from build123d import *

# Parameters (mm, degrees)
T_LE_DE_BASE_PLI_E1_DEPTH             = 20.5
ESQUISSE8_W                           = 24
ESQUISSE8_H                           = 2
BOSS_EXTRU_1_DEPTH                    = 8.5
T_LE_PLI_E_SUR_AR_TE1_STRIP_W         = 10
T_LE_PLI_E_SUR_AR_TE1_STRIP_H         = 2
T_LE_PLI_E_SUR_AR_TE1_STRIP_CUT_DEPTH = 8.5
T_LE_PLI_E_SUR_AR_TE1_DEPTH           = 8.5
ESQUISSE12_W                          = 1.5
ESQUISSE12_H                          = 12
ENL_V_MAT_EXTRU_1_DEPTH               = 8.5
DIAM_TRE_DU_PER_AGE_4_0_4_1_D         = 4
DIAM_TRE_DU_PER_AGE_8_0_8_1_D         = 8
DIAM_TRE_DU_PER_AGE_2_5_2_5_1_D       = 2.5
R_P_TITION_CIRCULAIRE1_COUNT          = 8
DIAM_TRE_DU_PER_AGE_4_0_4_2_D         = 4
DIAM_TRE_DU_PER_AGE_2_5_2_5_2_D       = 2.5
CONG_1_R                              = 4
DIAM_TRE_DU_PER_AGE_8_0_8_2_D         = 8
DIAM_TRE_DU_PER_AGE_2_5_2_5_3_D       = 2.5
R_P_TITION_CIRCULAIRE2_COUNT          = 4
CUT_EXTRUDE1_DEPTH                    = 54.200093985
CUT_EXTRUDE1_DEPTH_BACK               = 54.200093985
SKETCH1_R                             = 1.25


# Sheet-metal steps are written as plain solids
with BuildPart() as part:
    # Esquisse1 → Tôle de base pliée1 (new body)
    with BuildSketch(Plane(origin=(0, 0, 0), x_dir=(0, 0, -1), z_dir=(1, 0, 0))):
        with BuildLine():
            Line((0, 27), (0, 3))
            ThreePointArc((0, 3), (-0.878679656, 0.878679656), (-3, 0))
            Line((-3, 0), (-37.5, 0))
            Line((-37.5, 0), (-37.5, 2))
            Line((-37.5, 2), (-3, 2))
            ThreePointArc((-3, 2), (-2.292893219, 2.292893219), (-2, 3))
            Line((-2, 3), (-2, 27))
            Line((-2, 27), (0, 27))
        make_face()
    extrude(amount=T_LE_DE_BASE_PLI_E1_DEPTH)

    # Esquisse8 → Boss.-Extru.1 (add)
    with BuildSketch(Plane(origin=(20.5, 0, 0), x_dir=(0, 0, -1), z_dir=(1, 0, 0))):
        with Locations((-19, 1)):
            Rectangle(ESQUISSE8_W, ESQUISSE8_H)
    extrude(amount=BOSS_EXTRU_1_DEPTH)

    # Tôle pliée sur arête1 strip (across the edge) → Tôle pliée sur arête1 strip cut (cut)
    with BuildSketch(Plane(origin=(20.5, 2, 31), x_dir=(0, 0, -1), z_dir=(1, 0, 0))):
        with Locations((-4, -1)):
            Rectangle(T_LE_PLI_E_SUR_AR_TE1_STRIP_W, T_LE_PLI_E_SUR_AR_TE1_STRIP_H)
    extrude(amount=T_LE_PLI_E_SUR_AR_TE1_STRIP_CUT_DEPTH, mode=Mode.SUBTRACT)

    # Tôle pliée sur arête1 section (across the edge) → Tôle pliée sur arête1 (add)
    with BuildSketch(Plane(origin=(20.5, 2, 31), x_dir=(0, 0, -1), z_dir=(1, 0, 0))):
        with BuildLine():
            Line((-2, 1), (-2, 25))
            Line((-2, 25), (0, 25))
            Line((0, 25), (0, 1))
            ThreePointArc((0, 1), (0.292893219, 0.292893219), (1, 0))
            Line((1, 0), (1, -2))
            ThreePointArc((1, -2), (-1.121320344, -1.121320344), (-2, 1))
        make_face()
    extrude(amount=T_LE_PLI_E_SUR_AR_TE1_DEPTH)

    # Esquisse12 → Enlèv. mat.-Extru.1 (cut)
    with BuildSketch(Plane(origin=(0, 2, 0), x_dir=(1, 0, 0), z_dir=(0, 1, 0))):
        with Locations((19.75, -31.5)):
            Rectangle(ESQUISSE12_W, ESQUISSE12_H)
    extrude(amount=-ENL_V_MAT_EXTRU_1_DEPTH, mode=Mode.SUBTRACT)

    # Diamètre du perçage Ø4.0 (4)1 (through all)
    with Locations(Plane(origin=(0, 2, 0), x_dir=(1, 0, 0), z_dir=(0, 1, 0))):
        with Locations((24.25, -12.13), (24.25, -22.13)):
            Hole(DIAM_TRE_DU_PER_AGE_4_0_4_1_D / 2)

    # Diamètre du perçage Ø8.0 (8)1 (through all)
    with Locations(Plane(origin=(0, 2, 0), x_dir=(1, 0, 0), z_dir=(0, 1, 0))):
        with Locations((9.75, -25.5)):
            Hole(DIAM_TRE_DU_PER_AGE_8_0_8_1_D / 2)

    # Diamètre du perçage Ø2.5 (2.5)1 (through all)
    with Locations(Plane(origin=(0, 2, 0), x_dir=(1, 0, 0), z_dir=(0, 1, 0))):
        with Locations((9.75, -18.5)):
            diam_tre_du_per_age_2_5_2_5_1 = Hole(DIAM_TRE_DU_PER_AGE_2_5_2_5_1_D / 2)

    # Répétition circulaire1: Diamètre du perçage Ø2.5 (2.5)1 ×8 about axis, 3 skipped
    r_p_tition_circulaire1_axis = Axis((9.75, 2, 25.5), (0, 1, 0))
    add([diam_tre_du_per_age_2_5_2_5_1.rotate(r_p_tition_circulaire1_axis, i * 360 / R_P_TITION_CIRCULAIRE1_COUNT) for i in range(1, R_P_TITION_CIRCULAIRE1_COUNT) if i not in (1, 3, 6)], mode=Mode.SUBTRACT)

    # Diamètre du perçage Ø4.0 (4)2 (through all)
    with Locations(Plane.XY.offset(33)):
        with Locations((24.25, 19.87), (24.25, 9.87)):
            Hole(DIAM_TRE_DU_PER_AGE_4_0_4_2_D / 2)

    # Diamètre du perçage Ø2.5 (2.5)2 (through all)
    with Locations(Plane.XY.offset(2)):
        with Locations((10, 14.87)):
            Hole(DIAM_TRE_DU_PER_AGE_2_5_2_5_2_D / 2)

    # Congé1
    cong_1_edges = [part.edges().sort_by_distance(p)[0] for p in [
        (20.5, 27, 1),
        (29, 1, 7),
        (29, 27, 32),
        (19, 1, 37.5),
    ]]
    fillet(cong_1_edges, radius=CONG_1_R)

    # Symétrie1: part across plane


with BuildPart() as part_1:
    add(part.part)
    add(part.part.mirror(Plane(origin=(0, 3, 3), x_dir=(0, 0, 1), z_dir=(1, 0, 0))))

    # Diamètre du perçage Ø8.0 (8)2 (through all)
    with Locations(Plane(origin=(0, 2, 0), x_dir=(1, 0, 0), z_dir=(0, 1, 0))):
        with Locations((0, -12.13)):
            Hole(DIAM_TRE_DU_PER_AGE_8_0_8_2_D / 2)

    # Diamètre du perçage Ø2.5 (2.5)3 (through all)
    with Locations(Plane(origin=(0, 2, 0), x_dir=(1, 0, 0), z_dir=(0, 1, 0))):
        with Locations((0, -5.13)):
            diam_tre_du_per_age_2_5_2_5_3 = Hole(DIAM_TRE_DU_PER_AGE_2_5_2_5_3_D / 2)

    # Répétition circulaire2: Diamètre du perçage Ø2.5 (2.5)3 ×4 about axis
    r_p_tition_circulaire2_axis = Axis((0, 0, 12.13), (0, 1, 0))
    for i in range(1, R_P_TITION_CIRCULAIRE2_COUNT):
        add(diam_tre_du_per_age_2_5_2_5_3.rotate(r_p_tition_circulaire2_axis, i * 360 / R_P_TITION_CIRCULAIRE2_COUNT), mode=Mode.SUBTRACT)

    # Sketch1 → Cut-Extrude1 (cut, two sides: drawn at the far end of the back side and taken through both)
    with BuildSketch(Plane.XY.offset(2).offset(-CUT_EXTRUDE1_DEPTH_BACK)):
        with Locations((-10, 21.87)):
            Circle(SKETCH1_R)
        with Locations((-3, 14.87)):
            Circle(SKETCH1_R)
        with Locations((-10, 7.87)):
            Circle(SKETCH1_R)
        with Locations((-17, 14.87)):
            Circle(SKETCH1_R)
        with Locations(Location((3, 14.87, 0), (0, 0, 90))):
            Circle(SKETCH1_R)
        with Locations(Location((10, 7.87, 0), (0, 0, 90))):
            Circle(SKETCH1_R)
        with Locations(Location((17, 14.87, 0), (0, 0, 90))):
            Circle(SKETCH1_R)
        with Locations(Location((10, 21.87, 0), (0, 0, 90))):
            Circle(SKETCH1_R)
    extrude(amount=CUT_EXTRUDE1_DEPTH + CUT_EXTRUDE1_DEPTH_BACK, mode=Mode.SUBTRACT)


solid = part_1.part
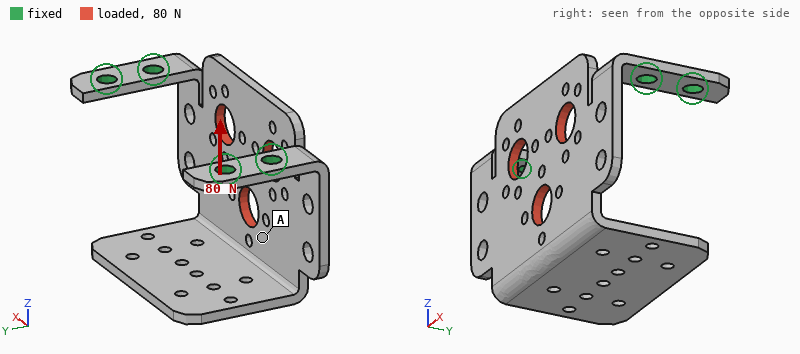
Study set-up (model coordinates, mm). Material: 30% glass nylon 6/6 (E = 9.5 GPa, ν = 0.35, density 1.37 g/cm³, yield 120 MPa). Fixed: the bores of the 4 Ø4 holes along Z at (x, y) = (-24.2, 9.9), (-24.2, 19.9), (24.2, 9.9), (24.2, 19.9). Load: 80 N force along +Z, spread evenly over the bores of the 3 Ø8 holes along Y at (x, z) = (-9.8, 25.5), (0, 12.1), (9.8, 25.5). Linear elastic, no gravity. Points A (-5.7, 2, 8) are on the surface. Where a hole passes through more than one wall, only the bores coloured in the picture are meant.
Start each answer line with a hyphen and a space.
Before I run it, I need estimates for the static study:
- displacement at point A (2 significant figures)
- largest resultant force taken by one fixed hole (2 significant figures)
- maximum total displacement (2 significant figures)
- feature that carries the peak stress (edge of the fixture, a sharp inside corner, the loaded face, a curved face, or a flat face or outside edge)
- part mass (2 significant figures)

- 0.49 mm
- 41 N
- 0.76 mm
- a flat face or outside edge
- 8.1 g
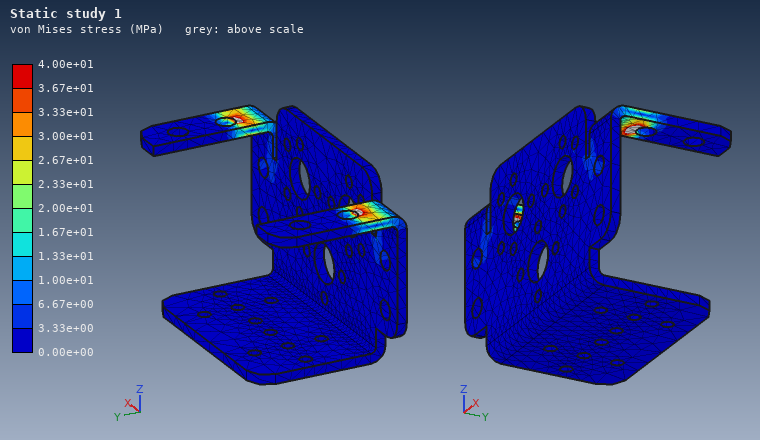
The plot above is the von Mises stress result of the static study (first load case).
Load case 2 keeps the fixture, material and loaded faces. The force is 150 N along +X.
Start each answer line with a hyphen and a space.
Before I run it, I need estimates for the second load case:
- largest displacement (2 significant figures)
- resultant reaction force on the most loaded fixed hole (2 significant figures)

- 0.30 mm
- 94 N
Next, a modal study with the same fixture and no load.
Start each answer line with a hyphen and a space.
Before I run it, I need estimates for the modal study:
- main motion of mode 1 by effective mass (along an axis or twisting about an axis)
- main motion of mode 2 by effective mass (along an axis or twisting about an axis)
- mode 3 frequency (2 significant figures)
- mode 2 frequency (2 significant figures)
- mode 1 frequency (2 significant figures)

- along Y
- along X
- 750 Hz
- 580 Hz
- 200 Hz
